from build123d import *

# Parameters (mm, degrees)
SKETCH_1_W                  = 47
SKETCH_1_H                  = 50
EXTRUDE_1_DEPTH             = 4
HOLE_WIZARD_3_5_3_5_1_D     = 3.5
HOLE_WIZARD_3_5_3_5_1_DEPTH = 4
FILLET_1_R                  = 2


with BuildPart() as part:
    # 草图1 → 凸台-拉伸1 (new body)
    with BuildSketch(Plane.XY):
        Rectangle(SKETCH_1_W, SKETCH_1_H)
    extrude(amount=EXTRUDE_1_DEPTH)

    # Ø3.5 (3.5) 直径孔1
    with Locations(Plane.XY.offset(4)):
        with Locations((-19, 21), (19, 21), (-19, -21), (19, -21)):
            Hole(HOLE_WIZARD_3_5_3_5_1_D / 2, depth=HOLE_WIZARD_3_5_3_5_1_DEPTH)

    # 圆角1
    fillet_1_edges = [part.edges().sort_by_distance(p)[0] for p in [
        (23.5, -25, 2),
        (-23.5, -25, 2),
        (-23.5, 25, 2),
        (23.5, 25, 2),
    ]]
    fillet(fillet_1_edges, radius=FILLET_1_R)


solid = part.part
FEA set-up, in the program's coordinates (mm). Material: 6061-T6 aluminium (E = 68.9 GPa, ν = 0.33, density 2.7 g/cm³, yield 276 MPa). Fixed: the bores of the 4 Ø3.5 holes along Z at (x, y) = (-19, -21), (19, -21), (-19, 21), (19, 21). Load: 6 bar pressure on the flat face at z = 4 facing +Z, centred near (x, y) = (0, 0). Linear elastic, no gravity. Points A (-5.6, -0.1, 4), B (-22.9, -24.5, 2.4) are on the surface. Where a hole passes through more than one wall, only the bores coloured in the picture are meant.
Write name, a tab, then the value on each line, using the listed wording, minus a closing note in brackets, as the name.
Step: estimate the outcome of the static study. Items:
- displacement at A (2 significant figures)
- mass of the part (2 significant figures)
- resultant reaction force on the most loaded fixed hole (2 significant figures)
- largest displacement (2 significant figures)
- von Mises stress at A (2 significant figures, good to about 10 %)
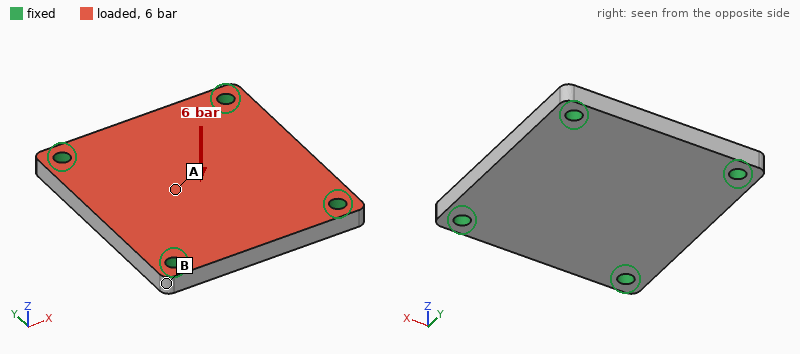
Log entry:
displacement at A	28 µm
mass of the part	25 g
resultant reaction force on the most loaded fixed hole	350 N
largest displacement	29 µm
von Mises stress at A	18 MPa
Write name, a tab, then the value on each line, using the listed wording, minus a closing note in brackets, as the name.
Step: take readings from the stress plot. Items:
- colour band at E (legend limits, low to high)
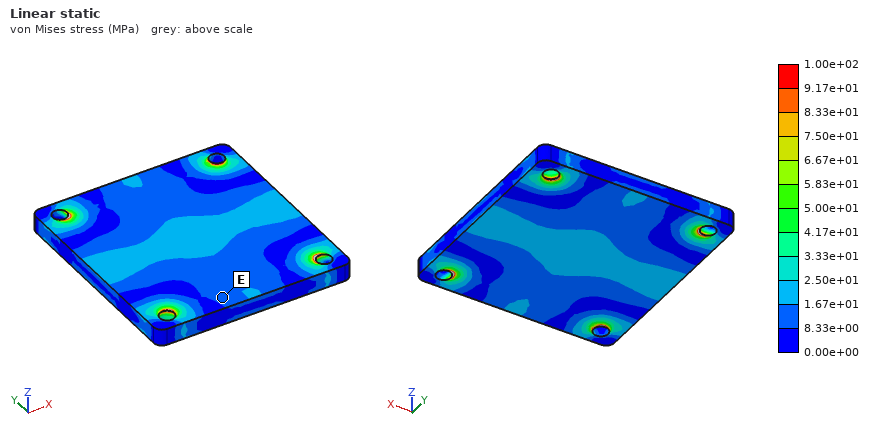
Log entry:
colour band at E	8.33e+00 to 1.67e+01 MPa
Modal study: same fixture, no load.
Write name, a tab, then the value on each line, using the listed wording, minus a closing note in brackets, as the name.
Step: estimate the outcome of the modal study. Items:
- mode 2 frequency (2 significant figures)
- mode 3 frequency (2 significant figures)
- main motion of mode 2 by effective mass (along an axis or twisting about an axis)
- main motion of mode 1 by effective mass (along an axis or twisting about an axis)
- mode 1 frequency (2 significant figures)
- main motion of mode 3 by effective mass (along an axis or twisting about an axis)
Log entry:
mode 2 frequency	13 kHz
mode 3 frequency	15 kHz
main motion of mode 2 by effective mass	twisting about Y
main motion of mode 1 by effective mass	along Z
mode 1 frequency	8400 Hz
main motion of mode 3 by effective mass	twisting about X
